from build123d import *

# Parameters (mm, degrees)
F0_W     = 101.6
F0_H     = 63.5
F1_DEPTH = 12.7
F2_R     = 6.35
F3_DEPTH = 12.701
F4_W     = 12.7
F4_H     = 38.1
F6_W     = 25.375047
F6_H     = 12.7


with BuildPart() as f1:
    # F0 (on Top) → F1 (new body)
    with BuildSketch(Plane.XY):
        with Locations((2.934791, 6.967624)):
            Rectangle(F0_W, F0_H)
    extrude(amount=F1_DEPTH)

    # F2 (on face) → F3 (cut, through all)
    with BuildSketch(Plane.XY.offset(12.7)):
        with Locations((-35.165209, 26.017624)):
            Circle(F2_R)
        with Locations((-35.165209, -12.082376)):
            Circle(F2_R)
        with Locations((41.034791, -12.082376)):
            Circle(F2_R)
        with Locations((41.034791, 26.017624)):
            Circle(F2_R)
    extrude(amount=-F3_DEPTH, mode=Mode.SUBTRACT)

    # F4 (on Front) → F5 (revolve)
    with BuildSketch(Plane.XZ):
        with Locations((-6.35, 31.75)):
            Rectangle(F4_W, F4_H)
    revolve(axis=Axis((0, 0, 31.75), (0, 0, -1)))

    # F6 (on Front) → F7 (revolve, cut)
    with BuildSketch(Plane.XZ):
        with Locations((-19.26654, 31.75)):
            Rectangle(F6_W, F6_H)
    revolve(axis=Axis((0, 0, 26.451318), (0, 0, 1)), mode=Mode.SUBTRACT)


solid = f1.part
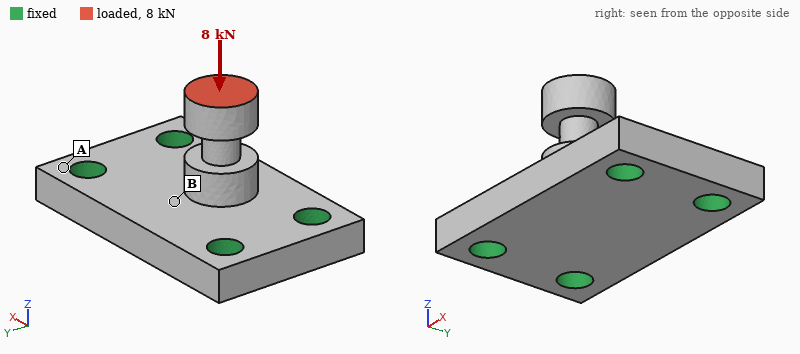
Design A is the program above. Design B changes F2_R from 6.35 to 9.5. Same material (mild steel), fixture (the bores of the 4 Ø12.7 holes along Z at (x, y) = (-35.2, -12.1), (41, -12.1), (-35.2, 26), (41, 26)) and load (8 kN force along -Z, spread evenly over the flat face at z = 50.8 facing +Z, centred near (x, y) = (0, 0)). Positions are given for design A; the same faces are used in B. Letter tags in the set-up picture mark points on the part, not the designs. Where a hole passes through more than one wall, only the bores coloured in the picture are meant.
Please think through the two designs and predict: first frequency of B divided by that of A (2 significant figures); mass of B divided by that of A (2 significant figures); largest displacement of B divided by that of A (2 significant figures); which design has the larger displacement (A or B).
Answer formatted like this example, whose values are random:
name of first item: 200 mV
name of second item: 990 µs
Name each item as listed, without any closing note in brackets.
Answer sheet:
first frequency of B divided by that of A: 1.0
mass of B divided by that of A: 0.91
largest displacement of B divided by that of A: 0.87
which design has the larger displacement: A
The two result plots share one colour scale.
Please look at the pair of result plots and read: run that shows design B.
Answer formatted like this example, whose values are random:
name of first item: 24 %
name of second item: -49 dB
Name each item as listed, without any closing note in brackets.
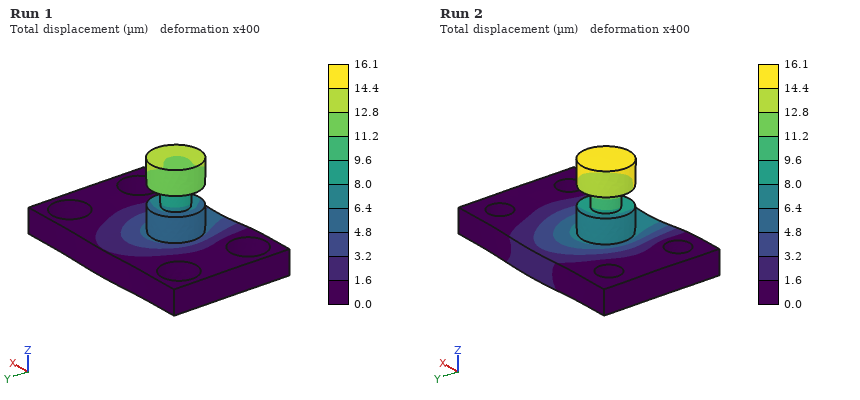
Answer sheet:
run that shows design B: Run 1
